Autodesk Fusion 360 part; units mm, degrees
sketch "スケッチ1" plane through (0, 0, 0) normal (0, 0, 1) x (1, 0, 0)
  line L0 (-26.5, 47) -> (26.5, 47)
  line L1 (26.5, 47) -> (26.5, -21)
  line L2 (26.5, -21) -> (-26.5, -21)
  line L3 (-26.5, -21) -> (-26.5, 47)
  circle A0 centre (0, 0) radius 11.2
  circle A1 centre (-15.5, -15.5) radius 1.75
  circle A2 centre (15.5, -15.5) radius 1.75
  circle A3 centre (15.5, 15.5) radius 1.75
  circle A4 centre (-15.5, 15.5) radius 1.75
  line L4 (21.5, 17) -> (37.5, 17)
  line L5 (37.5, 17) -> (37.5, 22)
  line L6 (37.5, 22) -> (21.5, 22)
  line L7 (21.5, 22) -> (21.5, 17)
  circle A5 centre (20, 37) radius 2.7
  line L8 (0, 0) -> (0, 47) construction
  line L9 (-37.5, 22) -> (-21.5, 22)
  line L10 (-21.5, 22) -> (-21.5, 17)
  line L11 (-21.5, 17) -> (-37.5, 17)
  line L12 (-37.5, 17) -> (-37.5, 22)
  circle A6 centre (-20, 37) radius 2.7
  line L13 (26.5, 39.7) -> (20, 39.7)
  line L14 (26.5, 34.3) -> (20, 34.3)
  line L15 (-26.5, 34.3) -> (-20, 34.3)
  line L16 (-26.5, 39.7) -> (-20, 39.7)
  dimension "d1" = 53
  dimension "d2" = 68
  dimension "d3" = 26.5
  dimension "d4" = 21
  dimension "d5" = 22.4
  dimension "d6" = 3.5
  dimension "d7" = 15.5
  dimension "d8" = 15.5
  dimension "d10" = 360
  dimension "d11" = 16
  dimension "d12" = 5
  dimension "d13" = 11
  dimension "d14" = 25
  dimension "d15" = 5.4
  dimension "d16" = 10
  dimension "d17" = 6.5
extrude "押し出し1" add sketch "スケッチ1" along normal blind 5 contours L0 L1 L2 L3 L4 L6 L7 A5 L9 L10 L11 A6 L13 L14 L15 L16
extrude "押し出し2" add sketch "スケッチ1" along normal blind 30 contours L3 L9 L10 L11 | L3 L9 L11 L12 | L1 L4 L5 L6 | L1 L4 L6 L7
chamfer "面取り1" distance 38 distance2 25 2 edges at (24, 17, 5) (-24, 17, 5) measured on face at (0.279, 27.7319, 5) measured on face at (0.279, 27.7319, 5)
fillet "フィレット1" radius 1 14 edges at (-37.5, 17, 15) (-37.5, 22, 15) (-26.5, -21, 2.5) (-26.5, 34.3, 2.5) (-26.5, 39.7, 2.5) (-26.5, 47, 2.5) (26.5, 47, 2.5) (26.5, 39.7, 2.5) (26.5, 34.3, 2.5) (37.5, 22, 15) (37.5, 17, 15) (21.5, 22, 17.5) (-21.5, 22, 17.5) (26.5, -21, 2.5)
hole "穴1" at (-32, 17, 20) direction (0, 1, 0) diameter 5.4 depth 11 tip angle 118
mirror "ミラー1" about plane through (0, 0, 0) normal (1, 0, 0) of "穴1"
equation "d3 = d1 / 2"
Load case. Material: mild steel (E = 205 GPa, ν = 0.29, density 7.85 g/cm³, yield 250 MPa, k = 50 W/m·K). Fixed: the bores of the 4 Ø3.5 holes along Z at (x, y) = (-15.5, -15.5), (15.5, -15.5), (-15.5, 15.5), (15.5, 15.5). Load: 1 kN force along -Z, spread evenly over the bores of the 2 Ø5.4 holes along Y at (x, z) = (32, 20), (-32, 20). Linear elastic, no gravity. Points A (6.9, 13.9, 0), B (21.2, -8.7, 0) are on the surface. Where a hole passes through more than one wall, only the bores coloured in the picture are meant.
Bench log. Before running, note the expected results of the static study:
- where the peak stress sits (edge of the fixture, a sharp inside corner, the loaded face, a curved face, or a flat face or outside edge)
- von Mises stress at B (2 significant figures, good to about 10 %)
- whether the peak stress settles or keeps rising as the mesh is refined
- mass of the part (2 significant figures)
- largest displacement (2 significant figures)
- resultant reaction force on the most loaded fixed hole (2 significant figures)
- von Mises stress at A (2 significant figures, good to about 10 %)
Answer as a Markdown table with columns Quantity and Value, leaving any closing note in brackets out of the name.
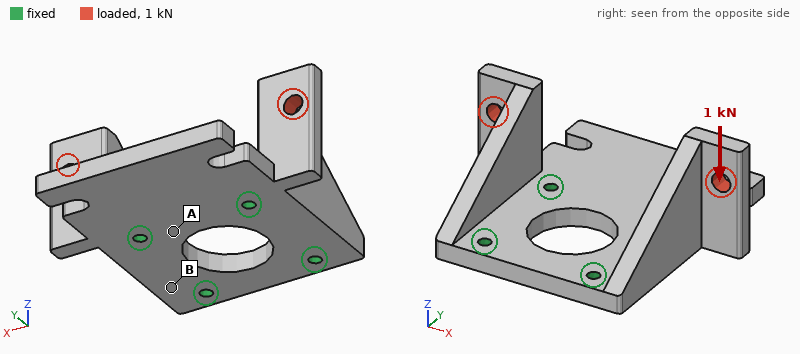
| Quantity | Value |
|---|---|
| where the peak stress sits | edge of the fixture |
| von Mises stress at B | 16 MPa |
| whether the peak stress settles or keeps rising as the mesh is refined | keeps rising |
| mass of the part | 190 g |
| largest displacement | 38 µm |
| resultant reaction force on the most loaded fixed hole | 530 N |
| von Mises stress at A | 7.1 MPa |
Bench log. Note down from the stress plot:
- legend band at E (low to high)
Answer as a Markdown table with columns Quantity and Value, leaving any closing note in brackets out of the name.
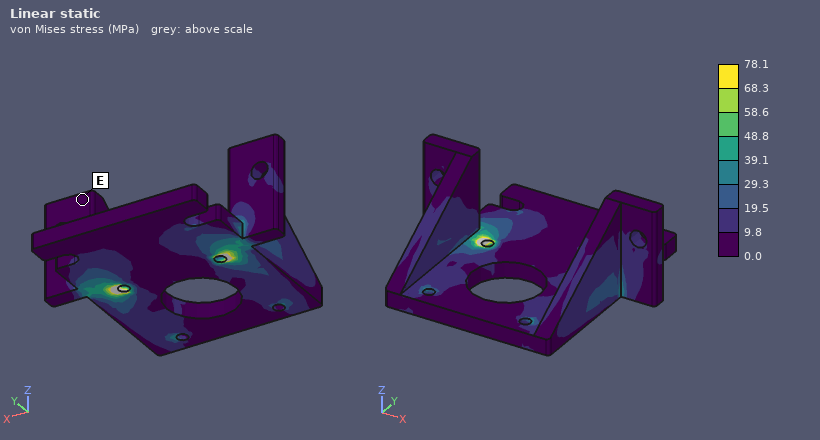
| Quantity | Value |
|---|---|
| legend band at E | 0.0 to 9.8 MPa |
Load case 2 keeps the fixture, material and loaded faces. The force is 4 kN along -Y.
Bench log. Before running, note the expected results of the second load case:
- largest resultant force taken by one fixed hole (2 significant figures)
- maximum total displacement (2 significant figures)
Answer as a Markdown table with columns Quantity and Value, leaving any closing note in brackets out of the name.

| Quantity | Value |
|---|---|
| largest resultant force taken by one fixed hole | 1.7 kN |
| maximum total displacement | 63 µm |
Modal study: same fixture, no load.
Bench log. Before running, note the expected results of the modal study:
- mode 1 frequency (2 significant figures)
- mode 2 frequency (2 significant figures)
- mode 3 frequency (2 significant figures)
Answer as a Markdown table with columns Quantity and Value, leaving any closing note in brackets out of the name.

| Quantity | Value |
|---|---|
| mode 1 frequency | 4000 Hz |
| mode 2 frequency | 4100 Hz |
| mode 3 frequency | 4100 Hz |
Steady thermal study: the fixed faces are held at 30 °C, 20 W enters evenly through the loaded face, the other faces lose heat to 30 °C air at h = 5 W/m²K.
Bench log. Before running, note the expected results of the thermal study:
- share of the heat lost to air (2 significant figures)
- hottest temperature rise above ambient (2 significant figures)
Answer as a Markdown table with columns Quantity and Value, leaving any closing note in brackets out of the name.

| Quantity | Value |
|---|---|
| share of the heat lost to air | 3.8 % |
| hottest temperature rise above ambient | 51 K |
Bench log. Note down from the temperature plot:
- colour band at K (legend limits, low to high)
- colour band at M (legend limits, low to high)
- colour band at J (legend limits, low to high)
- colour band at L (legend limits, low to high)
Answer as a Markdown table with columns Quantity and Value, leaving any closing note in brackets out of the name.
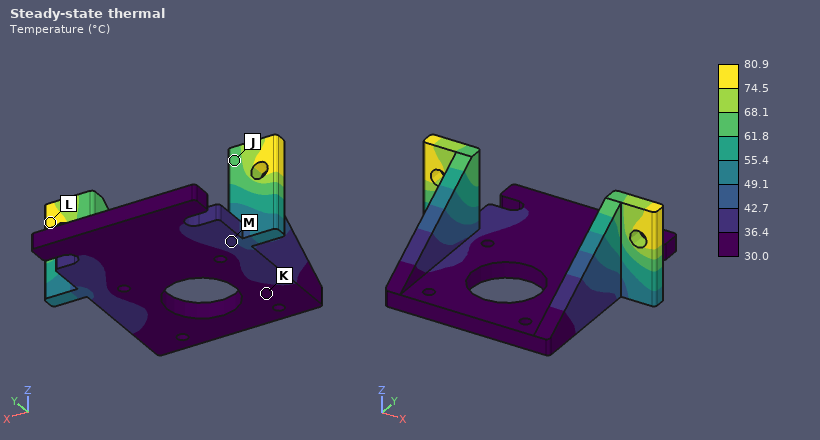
| Quantity | Value |
|---|---|
| colour band at K | 30.0 to 36.4 °C |
| colour band at M | 36.4 to 42.7 °C |
| colour band at J | 61.8 to 68.1 °C |
| colour band at L | 74.5 to 80.9 °C |
